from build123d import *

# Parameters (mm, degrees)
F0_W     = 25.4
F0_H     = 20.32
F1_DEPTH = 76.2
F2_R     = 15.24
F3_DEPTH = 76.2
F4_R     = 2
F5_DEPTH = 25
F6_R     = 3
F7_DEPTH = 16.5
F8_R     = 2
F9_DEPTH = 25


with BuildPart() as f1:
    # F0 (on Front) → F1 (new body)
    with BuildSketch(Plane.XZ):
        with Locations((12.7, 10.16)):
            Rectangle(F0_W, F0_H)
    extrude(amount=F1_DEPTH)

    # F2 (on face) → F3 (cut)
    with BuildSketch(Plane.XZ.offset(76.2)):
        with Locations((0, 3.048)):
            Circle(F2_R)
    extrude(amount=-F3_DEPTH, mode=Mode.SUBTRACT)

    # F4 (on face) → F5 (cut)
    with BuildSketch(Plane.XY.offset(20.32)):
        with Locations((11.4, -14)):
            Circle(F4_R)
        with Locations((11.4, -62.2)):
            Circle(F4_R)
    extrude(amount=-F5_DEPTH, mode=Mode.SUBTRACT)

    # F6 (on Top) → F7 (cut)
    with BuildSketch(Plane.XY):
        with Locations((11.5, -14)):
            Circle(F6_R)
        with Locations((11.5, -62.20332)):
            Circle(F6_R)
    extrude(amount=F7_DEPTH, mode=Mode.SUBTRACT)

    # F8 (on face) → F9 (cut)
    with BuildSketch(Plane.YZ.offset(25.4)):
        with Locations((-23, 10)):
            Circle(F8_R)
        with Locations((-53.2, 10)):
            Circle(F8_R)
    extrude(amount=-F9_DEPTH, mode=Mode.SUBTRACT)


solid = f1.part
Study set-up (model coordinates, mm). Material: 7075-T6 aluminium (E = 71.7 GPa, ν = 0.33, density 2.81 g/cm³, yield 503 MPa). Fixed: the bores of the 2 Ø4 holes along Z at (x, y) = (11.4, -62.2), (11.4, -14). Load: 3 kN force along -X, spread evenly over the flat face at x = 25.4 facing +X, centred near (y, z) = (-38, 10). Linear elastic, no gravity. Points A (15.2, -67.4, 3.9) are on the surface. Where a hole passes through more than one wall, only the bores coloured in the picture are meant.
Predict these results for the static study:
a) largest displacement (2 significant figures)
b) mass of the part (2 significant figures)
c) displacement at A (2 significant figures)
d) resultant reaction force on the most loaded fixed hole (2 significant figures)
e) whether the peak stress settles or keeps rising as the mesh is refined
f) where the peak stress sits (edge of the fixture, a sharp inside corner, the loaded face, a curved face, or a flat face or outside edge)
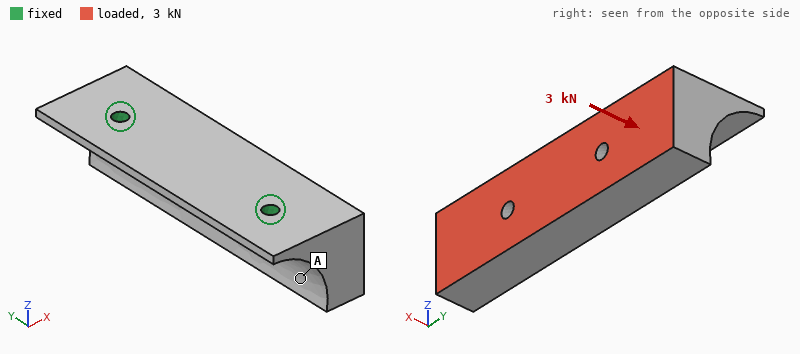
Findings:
97 µm
60 g
59 µm
1.5 kN
keeps rising
edge of the fixture
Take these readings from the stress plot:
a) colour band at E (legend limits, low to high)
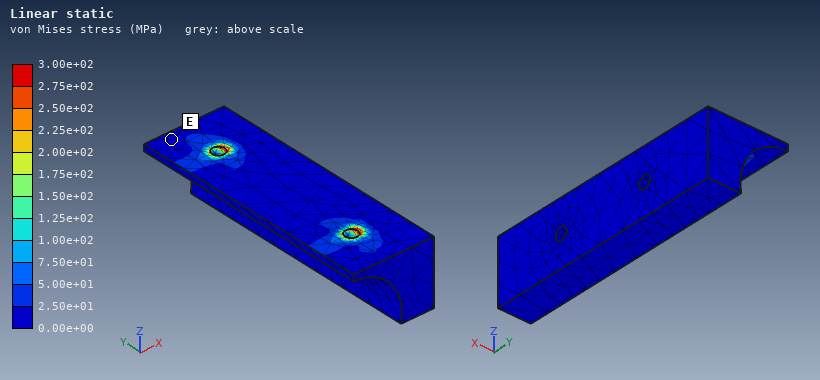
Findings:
0.00e+00 to 2.50e+01 MPa
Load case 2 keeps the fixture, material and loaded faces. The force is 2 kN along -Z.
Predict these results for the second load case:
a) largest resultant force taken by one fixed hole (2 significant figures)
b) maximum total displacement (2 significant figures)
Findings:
1.0 kN
0.10 mm
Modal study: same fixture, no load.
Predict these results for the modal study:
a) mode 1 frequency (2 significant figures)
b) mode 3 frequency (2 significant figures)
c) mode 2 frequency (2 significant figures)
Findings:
4300 Hz
13 kHz
9100 Hz
